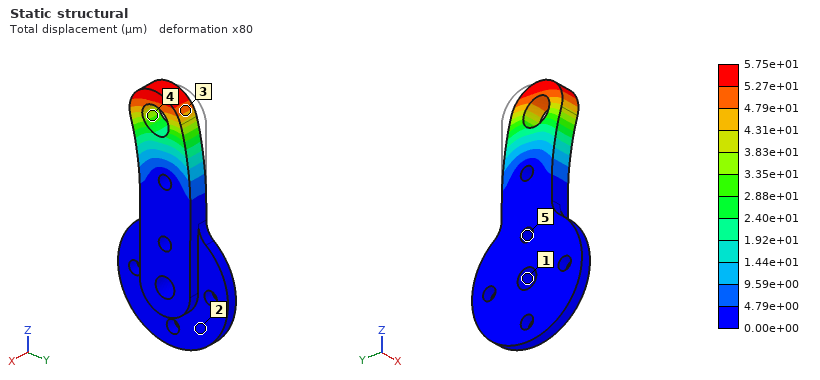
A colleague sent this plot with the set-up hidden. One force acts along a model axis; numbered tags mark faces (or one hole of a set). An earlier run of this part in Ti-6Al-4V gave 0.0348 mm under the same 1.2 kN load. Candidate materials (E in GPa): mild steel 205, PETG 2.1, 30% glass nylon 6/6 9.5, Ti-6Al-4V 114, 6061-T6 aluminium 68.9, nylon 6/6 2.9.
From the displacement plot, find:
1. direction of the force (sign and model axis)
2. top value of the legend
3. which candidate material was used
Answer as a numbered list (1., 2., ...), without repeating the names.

1. -Y
2. 5.75e+01 µm
3. 6061-T6 aluminium
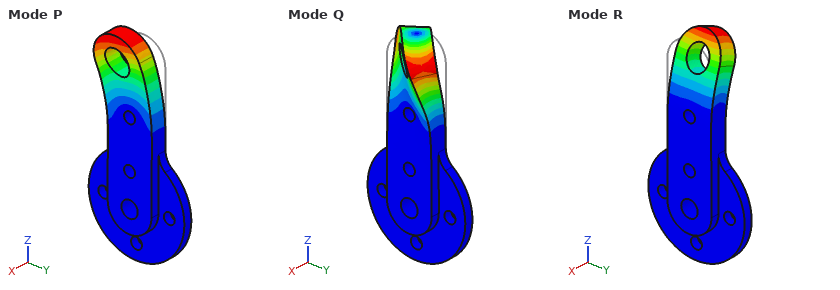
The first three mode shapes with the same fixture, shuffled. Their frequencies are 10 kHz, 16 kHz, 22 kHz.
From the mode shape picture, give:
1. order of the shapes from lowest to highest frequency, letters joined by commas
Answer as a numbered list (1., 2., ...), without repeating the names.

1. R, P, Q
